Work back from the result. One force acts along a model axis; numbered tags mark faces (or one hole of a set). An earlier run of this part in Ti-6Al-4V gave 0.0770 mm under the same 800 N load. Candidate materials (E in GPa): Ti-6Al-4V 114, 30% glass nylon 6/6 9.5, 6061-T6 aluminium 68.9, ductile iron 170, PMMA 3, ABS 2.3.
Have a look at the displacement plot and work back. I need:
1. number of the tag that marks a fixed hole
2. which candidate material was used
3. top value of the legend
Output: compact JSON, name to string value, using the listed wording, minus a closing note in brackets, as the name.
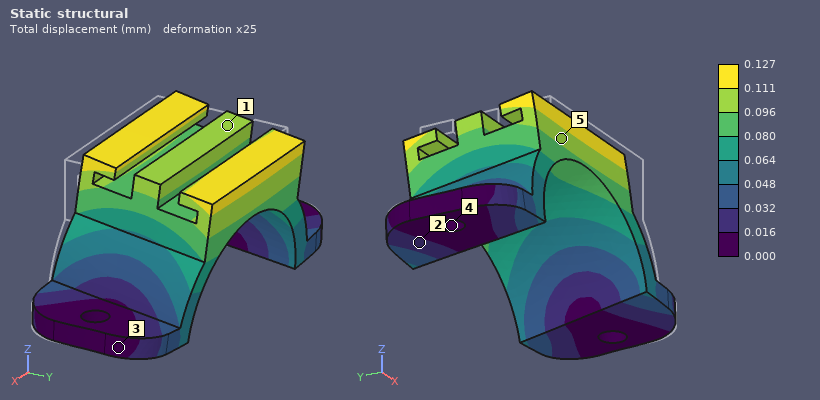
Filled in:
{"number of the tag that marks a fixed hole": "4", "which candidate material was used": "6061-T6 aluminium", "top value of the legend": "0.127 mm"}
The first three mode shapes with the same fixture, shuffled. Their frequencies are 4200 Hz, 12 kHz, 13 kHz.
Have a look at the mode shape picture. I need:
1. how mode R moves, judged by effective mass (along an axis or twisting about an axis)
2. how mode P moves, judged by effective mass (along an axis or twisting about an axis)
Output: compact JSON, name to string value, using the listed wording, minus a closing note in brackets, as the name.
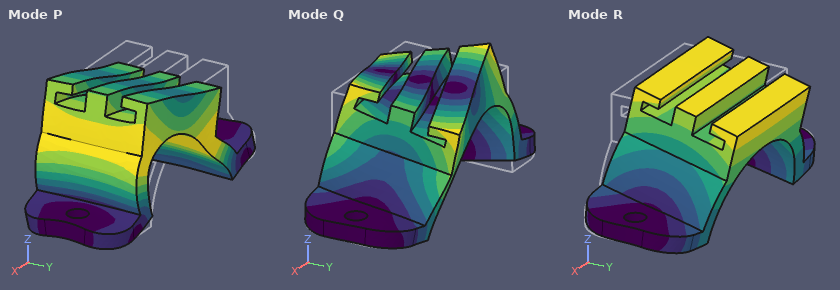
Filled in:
{"how mode R moves, judged by effective mass": "along Y", "how mode P moves, judged by effective mass": "along X"}
